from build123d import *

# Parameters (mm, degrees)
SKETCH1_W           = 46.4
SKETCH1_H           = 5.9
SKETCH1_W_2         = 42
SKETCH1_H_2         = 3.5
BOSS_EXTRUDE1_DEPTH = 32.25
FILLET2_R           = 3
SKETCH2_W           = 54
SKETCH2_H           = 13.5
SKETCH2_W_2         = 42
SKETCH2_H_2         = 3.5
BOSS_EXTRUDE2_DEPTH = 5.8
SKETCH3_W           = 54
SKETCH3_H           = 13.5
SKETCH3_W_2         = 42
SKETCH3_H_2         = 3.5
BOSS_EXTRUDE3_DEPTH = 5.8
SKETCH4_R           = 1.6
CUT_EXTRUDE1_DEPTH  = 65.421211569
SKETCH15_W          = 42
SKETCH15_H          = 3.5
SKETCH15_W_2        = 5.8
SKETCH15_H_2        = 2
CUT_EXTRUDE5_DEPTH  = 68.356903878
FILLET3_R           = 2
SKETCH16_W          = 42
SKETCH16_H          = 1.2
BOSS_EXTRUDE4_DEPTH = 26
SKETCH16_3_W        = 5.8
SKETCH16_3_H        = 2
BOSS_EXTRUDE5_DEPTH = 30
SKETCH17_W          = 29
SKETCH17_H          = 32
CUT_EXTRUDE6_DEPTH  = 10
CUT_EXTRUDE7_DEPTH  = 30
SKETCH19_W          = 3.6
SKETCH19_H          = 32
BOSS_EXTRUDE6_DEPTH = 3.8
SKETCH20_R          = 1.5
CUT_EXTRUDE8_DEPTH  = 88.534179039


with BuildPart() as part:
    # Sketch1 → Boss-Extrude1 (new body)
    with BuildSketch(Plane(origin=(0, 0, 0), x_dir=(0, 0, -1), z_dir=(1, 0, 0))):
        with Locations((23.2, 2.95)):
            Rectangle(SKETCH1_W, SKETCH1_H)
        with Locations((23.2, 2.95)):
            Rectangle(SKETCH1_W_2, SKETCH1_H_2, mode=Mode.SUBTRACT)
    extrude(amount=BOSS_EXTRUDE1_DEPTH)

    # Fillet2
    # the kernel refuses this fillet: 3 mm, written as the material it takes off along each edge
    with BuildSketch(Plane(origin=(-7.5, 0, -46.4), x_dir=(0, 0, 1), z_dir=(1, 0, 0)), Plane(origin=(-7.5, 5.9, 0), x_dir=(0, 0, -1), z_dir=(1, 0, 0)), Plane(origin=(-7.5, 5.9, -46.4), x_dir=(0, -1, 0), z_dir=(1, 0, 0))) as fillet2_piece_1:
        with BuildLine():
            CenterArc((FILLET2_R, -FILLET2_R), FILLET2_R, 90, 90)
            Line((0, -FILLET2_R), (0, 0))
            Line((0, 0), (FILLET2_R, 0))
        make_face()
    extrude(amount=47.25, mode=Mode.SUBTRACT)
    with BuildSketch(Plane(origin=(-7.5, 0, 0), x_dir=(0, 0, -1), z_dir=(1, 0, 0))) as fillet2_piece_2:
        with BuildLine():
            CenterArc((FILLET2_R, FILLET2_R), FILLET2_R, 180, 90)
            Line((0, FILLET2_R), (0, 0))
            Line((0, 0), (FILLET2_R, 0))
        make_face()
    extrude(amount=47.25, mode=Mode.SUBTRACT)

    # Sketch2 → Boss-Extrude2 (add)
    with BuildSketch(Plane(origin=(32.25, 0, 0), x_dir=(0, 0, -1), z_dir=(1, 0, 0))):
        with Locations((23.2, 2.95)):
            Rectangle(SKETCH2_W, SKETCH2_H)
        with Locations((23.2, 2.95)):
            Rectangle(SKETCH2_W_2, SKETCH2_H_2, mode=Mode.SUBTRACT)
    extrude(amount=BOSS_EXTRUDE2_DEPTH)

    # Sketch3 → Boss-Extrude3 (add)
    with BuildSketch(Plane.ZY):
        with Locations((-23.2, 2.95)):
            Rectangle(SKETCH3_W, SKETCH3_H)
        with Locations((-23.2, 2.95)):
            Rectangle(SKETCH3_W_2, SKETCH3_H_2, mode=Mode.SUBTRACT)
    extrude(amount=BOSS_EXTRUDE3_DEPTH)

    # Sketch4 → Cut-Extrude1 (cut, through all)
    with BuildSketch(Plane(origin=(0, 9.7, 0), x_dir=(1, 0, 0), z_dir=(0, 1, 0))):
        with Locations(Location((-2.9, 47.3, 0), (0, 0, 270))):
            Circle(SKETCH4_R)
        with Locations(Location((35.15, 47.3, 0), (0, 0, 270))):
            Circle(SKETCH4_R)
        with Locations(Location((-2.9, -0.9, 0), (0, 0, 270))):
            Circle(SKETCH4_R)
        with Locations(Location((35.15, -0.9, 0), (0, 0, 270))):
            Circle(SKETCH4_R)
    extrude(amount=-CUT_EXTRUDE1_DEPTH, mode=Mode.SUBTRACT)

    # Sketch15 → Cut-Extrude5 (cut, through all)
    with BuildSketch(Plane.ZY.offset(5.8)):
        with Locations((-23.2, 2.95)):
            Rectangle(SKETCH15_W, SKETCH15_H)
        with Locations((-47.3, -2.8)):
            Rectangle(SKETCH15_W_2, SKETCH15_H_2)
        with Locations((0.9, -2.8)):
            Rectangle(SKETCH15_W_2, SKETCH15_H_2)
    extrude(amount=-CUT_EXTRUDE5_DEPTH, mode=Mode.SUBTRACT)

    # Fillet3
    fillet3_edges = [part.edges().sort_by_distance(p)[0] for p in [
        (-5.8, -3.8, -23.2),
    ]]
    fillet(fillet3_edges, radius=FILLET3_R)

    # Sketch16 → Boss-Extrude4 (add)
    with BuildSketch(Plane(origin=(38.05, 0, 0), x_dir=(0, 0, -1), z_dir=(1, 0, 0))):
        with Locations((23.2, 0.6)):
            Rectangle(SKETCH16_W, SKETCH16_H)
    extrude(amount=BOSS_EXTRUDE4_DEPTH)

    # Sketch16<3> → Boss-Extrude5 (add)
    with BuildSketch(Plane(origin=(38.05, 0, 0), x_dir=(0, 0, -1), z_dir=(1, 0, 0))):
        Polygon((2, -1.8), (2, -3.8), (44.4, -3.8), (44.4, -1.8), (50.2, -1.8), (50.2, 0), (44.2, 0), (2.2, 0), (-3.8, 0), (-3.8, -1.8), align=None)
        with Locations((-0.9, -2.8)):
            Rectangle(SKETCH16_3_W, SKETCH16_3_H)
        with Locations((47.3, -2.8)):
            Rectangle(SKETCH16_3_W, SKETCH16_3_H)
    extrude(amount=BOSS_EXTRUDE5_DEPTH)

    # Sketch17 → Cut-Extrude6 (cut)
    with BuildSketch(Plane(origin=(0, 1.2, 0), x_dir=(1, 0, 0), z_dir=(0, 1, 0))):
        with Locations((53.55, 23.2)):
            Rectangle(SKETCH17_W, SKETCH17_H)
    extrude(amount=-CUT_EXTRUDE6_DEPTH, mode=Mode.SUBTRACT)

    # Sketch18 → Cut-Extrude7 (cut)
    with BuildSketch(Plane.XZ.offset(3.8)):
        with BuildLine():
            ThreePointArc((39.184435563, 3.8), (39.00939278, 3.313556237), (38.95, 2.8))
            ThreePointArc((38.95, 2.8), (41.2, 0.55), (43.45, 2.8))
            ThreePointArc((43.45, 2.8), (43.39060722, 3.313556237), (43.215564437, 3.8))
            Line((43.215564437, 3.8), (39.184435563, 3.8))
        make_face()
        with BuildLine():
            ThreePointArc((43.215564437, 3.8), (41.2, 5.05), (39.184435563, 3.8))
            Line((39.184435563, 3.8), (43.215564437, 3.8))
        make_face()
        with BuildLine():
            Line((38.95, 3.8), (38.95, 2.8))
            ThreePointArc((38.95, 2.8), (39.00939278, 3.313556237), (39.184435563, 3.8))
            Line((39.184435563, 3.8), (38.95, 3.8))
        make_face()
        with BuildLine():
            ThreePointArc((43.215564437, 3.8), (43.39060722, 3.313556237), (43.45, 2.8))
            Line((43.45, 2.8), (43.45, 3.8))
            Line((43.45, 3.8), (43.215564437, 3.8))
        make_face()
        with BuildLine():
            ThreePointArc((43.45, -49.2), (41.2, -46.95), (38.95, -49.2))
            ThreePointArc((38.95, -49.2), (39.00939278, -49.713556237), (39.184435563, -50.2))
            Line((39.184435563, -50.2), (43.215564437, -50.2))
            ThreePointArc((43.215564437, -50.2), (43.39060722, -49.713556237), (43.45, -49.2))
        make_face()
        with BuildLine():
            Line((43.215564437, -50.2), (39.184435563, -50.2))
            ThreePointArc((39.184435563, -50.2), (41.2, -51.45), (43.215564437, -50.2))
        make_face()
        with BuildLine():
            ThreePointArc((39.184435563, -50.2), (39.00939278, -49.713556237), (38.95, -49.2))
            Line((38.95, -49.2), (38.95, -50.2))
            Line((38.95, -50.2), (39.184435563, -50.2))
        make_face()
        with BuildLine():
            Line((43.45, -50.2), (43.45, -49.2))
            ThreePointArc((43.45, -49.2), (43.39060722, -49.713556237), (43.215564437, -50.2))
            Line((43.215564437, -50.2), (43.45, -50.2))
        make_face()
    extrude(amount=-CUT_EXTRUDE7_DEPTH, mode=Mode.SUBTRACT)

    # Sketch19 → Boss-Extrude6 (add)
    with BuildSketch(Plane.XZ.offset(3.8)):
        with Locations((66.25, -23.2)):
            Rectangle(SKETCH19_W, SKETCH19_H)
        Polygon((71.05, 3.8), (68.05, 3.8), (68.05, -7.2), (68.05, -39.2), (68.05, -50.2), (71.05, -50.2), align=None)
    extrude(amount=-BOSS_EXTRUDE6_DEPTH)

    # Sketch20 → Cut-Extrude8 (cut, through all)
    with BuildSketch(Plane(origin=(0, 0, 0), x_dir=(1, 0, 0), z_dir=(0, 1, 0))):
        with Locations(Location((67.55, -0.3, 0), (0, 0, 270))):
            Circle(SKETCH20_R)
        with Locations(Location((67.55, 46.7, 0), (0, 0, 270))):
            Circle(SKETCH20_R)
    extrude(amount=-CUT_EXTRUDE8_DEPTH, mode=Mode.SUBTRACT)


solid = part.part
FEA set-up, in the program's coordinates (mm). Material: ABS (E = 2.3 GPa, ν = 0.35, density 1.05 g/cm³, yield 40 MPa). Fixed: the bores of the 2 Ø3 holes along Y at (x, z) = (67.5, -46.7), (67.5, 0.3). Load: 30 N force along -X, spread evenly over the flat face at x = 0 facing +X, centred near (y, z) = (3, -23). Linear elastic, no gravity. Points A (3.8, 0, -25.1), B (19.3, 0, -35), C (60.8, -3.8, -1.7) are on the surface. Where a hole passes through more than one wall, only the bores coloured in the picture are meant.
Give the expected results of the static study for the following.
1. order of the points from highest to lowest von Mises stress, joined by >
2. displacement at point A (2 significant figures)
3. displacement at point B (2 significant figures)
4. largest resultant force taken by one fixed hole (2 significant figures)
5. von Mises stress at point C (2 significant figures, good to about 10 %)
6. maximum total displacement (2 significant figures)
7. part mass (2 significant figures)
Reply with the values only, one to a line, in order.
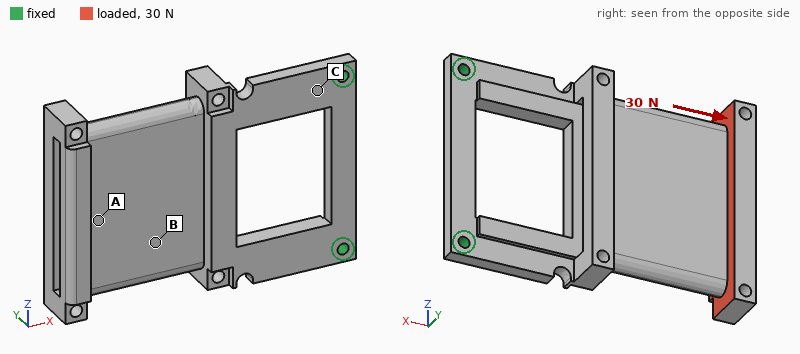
C > A > B
0.80 mm
0.52 mm
15 N
1.7 MPa
0.99 mm
14 g
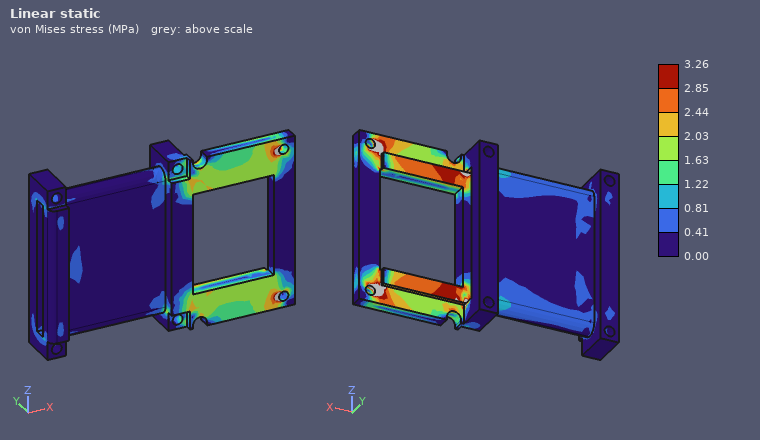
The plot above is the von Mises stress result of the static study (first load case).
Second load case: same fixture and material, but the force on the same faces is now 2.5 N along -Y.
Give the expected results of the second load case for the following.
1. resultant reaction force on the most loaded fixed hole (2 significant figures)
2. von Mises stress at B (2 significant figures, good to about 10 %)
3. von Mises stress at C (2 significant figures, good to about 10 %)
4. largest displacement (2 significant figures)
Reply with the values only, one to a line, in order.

1.4 N
0.34 MPa
2.2 MPa
0.97 mm
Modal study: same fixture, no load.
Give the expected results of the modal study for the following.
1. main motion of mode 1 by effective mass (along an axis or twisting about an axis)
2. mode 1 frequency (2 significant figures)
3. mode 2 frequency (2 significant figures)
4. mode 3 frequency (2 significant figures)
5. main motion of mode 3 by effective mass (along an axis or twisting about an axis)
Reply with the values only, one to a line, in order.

along Y
110 Hz
500 Hz
670 Hz
along Y
